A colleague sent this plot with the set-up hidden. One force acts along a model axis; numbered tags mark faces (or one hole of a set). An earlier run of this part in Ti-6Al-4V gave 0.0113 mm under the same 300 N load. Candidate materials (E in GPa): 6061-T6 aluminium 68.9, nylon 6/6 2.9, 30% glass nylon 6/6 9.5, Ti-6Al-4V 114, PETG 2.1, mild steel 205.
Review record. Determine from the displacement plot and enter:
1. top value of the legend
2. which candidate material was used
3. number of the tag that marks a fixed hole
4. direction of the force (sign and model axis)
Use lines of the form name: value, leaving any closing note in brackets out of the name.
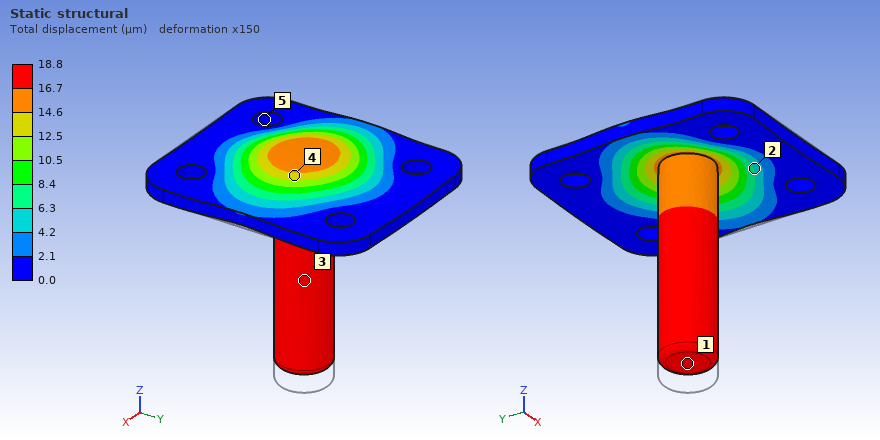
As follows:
top value of the legend: 18.8 µm
which candidate material was used: 6061-T6 aluminium
number of the tag that marks a fixed hole: 5
direction of the force: +Z
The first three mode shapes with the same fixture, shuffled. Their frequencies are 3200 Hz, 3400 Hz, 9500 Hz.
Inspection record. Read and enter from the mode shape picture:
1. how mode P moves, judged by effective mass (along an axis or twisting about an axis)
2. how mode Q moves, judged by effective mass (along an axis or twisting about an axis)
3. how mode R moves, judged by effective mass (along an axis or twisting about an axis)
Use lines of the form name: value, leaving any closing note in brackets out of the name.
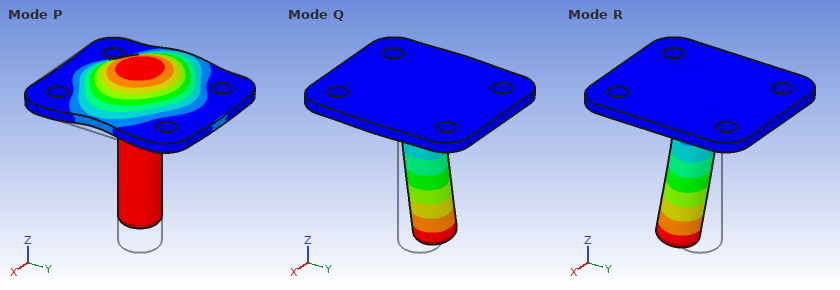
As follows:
how mode P moves, judged by effective mass: along Z
how mode Q moves, judged by effective mass: along X
how mode R moves, judged by effective mass: along Y
